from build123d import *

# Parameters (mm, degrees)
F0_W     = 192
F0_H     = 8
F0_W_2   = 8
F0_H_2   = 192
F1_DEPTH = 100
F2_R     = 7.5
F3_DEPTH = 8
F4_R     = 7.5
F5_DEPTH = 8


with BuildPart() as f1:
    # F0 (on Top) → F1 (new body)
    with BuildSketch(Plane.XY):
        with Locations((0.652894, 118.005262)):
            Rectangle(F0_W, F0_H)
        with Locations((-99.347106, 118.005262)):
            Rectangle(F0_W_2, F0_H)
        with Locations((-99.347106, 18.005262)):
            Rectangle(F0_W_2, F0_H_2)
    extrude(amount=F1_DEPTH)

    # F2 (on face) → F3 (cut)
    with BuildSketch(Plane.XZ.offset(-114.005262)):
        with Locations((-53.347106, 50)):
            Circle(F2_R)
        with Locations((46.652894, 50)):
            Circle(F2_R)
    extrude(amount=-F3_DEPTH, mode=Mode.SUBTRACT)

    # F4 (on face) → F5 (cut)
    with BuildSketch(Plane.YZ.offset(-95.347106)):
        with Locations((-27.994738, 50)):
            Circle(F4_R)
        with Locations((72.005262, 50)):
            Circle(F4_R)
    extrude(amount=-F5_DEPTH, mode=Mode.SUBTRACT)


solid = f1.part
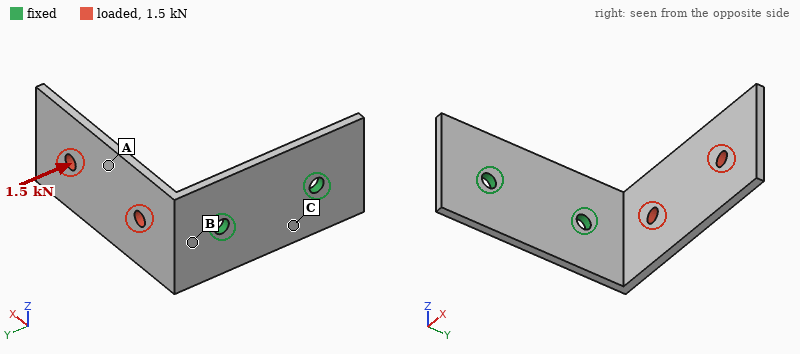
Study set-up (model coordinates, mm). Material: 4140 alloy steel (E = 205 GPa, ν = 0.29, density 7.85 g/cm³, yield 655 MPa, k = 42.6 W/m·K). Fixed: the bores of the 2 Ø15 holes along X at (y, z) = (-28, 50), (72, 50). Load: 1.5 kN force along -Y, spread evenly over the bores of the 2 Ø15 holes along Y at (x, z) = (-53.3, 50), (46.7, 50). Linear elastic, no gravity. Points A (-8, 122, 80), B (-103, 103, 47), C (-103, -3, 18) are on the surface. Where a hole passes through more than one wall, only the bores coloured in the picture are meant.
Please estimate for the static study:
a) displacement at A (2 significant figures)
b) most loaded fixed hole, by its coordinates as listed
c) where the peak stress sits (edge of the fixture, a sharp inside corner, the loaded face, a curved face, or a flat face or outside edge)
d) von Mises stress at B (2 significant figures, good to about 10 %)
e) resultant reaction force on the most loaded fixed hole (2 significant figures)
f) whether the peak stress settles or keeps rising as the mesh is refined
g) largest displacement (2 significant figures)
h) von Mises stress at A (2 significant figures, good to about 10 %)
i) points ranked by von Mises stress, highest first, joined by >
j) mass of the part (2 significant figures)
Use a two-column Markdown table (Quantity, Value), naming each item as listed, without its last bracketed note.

| Quantity | Value |
|---|---|
| displacement at A | 1.1 mm |
| most loaded fixed hole, by its coordinates as listed | (72, 50) |
| where the peak stress sits | edge of the fixture |
| von Mises stress at B | 120 MPa |
| resultant reaction force on the most loaded fixed hole | 1.4 kN |
| whether the peak stress settles or keeps rising as the mesh is refined | keeps rising |
| largest displacement | 2.9 mm |
| von Mises stress at A | 39 MPa |
| points ranked by von Mises stress, highest first, joined by > | B > A > C |
| mass of the part | 2.4 kg |
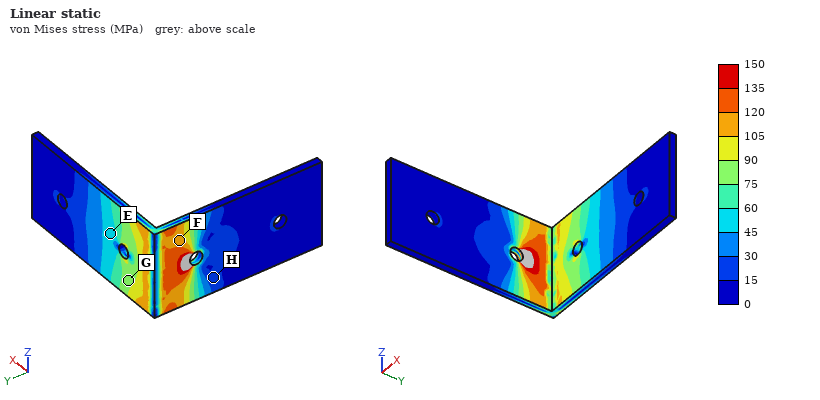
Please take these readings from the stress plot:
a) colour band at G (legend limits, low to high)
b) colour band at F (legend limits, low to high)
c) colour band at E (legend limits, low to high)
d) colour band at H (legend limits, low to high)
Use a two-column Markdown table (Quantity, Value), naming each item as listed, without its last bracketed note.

| Quantity | Value |
|---|---|
| colour band at G | 75 to 90 MPa |
| colour band at F | 105 to 120 MPa |
| colour band at E | 45 to 60 MPa |
| colour band at H | 15 to 30 MPa |
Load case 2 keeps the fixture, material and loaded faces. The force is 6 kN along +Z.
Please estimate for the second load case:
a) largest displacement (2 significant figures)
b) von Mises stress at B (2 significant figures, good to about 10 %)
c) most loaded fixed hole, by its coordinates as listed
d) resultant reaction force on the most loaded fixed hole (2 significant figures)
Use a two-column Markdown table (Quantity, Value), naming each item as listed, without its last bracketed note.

| Quantity | Value |
|---|---|
| largest displacement | 3.2 mm |
| von Mises stress at B | 350 MPa |
| most loaded fixed hole, by its coordinates as listed | (72, 50) |
| resultant reaction force on the most loaded fixed hole | 8.2 kN |
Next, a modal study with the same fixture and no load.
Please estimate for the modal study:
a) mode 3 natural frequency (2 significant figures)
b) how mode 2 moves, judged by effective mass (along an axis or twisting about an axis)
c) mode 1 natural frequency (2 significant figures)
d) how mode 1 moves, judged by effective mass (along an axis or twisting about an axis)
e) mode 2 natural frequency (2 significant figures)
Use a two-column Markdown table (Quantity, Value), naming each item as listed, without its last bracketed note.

| Quantity | Value |
|---|---|
| mode 3 natural frequency | 680 Hz |
| how mode 2 moves, judged by effective mass | along Z |
| mode 1 natural frequency | 130 Hz |
| how mode 1 moves, judged by effective mass | along Y |
| mode 2 natural frequency | 230 Hz |
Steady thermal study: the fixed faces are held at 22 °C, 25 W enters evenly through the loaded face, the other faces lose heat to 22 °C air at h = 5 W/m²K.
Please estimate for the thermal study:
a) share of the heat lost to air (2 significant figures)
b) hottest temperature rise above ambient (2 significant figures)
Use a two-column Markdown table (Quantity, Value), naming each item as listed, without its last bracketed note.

| Quantity | Value |
|---|---|
| share of the heat lost to air | 45 % |
| hottest temperature rise above ambient | 67 K |
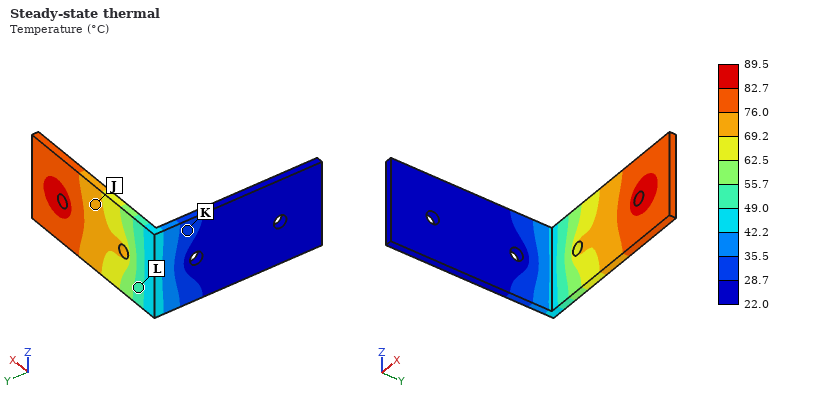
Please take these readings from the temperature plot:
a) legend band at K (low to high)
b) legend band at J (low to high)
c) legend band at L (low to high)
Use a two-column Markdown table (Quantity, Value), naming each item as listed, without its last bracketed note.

| Quantity | Value |
|---|---|
| legend band at K | 28.7 to 35.5 °C |
| legend band at J | 69.2 to 76.0 °C |
| legend band at L | 49.0 to 55.7 °C |
